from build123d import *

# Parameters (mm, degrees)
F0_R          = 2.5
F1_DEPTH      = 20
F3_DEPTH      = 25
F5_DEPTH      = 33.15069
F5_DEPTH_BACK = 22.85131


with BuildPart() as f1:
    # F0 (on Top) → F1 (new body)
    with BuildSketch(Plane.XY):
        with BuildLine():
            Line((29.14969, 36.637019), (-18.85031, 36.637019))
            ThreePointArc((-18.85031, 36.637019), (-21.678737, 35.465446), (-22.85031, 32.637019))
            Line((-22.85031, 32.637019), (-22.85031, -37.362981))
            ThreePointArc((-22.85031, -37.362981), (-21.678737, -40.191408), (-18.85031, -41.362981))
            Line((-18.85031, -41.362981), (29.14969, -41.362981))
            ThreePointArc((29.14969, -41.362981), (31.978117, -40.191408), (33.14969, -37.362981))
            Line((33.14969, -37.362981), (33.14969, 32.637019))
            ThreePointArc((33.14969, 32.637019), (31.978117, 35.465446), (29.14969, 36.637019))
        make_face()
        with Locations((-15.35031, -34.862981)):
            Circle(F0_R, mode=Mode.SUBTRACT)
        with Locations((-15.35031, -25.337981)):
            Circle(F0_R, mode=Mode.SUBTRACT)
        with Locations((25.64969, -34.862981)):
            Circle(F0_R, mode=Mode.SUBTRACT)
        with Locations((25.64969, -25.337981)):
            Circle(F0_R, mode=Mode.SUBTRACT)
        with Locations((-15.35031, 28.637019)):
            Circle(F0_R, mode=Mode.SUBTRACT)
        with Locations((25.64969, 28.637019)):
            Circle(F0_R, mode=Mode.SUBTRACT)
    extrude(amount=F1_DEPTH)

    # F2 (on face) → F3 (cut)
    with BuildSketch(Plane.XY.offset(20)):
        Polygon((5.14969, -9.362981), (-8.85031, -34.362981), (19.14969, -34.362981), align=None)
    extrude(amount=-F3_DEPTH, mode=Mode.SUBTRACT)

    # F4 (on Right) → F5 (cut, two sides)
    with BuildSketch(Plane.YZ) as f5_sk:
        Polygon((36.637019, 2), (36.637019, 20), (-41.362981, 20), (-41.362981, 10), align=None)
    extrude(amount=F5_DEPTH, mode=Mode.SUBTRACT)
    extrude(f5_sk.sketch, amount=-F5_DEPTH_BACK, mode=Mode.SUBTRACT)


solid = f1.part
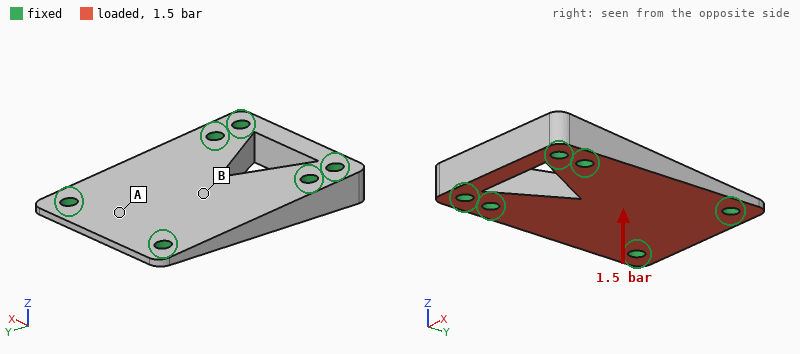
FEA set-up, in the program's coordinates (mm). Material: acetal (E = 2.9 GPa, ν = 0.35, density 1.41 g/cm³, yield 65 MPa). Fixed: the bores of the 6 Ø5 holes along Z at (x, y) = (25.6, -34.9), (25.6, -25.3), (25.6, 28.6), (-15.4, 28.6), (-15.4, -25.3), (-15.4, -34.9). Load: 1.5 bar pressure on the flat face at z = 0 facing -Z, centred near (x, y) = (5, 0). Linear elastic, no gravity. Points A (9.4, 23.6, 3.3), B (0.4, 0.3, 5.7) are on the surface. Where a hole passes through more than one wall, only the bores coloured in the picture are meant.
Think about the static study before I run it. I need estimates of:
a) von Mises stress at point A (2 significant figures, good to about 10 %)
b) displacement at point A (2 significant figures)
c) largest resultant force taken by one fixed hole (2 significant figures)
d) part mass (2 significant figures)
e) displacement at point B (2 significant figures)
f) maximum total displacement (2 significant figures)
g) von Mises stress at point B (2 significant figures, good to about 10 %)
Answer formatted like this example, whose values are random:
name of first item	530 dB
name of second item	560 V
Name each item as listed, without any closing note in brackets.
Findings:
von Mises stress at point A	5.5 MPa
displacement at point A	0.16 mm
largest resultant force taken by one fixed hole	160 N
part mass	32 g
displacement at point B	0.13 mm
maximum total displacement	0.20 mm
von Mises stress at point B	2.4 MPa
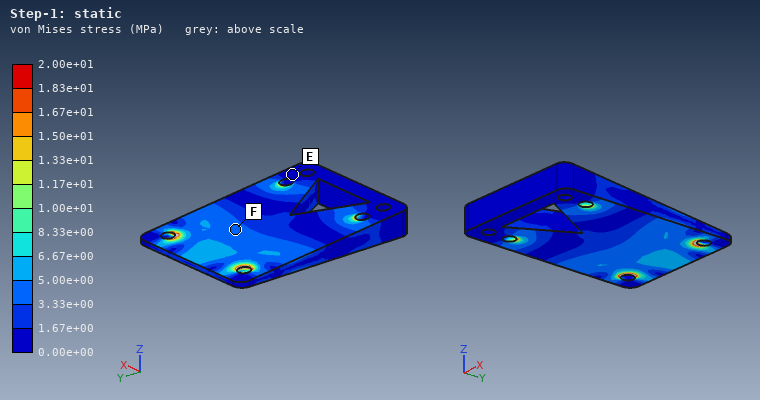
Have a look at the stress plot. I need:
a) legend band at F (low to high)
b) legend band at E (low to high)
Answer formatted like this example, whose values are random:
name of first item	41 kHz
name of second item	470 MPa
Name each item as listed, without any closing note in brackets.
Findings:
legend band at F	3.33e+00 to 5.00e+00 MPa
legend band at E	0.00e+00 to 1.67e+00 MPa
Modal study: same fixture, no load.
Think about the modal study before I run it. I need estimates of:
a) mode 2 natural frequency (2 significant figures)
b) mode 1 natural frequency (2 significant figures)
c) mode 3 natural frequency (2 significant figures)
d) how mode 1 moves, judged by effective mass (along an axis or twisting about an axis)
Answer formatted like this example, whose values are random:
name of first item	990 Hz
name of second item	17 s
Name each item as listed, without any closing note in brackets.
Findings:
mode 2 natural frequency	3000 Hz
mode 1 natural frequency	2200 Hz
mode 3 natural frequency	3200 Hz
how mode 1 moves, judged by effective mass	along Z
